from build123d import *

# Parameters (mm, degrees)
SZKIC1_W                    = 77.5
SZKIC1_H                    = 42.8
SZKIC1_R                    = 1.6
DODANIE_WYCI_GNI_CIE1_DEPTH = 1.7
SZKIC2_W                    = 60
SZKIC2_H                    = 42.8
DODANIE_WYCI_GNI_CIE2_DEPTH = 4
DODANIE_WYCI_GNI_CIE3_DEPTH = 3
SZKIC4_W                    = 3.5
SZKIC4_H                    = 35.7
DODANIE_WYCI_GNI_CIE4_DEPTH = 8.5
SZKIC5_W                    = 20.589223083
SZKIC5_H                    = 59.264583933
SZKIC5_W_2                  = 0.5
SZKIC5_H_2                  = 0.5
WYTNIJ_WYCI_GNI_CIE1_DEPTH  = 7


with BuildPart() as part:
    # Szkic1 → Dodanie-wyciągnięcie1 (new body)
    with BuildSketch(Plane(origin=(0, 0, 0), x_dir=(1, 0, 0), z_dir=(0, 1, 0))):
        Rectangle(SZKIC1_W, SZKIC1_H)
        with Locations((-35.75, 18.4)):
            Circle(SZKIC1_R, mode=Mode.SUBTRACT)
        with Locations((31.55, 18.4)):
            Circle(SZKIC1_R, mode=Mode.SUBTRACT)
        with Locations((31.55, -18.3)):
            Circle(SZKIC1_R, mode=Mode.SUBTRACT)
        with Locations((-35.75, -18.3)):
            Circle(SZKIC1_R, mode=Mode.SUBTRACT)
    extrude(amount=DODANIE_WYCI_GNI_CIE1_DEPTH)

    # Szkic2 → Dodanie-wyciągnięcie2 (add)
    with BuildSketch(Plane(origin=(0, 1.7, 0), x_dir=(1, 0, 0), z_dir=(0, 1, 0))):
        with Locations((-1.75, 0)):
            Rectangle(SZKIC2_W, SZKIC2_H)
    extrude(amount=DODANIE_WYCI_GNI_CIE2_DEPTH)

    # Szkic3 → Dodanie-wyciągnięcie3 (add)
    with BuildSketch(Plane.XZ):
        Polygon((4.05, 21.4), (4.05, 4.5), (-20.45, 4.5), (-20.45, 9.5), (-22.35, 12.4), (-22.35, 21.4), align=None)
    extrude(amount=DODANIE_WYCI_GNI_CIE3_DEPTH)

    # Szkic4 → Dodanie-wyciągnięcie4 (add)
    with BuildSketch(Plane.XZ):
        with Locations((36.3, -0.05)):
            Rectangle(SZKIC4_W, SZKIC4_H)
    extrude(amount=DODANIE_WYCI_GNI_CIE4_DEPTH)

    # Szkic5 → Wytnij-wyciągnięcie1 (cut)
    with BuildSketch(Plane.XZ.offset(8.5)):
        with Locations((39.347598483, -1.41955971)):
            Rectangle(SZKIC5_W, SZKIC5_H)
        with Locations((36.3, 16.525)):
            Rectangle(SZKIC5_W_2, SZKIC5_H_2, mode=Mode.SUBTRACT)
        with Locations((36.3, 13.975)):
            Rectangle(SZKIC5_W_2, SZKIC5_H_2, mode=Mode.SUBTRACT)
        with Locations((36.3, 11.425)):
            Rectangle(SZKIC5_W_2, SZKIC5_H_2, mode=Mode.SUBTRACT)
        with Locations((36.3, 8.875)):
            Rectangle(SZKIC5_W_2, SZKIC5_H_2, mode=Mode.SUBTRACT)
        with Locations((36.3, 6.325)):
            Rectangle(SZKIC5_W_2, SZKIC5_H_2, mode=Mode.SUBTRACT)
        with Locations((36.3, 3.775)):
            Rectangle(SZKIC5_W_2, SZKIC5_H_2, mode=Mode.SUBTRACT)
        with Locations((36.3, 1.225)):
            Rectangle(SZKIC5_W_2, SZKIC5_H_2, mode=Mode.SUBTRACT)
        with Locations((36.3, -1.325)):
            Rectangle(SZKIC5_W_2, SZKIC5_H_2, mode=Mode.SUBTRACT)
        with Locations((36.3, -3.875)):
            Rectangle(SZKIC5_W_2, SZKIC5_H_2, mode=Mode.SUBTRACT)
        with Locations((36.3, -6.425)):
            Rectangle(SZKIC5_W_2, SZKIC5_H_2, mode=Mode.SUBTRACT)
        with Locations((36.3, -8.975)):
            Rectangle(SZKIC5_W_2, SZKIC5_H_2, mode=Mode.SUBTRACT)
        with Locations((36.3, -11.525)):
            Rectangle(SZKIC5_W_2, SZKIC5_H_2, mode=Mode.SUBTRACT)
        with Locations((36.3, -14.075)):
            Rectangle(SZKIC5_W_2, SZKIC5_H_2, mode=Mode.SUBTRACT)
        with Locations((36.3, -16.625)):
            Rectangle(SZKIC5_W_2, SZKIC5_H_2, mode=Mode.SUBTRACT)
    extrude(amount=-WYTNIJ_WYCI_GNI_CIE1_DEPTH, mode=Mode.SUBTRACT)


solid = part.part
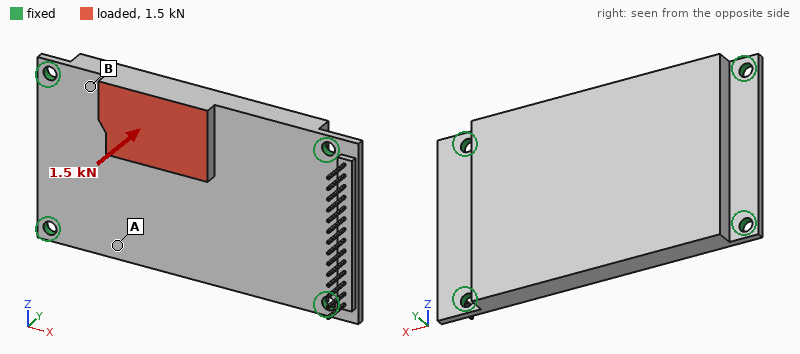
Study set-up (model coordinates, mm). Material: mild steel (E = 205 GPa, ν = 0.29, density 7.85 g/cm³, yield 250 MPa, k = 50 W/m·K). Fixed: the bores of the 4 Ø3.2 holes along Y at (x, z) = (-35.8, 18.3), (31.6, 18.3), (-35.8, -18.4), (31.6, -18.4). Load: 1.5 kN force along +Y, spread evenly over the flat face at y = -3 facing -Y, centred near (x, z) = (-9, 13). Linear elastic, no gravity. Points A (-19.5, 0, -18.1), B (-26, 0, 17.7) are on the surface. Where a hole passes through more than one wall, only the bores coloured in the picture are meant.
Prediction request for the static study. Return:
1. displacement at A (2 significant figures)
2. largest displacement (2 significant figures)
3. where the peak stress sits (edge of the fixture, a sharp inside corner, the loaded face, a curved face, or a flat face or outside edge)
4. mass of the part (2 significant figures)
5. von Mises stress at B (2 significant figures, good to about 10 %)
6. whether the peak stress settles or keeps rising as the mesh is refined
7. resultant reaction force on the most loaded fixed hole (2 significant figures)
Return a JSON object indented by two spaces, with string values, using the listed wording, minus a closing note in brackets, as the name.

{
  "displacement at A": "10 µm",
  "largest displacement": "45 µm",
  "where the peak stress sits": "edge of the fixture",
  "mass of the part": "140 g",
  "von Mises stress at B": "47 MPa",
  "whether the peak stress settles or keeps rising as the mesh is refined": "keeps rising",
  "resultant reaction force on the most loaded fixed hole": "1.2 kN"
}
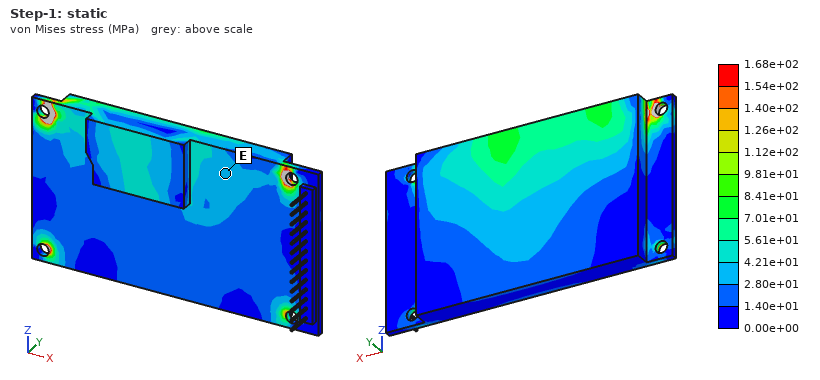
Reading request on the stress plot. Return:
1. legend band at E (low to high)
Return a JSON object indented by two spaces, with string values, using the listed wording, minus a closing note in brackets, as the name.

{
  "legend band at E": "2.80e+01 to 4.21e+01 MPa"
}
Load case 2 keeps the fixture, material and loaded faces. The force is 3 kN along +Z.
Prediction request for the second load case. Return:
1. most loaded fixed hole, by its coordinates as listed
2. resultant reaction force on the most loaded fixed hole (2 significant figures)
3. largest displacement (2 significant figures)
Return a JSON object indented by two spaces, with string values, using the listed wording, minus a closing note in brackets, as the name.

{
  "most loaded fixed hole, by its coordinates as listed": "(-35.8, 18.3)",
  "resultant reaction force on the most loaded fixed hole": "1.0 kN",
  "largest displacement": "25 µm"
}
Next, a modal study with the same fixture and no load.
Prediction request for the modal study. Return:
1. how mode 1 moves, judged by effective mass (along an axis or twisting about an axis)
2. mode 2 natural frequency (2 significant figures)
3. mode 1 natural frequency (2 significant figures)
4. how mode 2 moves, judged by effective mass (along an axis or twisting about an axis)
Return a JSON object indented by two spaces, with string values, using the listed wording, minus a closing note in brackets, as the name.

{
  "how mode 1 moves, judged by effective mass": "along Y",
  "mode 2 natural frequency": "6500 Hz",
  "mode 1 natural frequency": "3900 Hz",
  "how mode 2 moves, judged by effective mass": "twisting about X"
}
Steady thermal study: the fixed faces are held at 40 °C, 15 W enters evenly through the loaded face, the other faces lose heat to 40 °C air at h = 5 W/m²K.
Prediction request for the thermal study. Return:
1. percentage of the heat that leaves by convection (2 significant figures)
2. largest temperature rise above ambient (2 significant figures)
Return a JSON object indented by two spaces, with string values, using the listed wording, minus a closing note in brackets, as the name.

{
  "percentage of the heat that leaves by convection": "5.8 %",
  "largest temperature rise above ambient": "41 K"
}
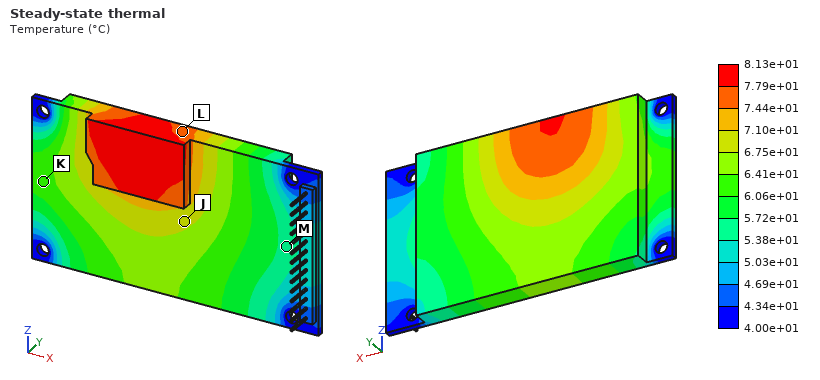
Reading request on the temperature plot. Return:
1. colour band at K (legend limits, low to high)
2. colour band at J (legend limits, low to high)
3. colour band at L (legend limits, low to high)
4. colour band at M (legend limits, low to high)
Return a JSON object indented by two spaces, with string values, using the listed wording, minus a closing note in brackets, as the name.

{
  "colour band at K": "6.06e+01 to 6.41e+01 °C",
  "colour band at J": "6.75e+01 to 7.10e+01 °C",
  "colour band at L": "7.44e+01 to 7.79e+01 °C",
  "colour band at M": "5.38e+01 to 5.72e+01 °C"
}
